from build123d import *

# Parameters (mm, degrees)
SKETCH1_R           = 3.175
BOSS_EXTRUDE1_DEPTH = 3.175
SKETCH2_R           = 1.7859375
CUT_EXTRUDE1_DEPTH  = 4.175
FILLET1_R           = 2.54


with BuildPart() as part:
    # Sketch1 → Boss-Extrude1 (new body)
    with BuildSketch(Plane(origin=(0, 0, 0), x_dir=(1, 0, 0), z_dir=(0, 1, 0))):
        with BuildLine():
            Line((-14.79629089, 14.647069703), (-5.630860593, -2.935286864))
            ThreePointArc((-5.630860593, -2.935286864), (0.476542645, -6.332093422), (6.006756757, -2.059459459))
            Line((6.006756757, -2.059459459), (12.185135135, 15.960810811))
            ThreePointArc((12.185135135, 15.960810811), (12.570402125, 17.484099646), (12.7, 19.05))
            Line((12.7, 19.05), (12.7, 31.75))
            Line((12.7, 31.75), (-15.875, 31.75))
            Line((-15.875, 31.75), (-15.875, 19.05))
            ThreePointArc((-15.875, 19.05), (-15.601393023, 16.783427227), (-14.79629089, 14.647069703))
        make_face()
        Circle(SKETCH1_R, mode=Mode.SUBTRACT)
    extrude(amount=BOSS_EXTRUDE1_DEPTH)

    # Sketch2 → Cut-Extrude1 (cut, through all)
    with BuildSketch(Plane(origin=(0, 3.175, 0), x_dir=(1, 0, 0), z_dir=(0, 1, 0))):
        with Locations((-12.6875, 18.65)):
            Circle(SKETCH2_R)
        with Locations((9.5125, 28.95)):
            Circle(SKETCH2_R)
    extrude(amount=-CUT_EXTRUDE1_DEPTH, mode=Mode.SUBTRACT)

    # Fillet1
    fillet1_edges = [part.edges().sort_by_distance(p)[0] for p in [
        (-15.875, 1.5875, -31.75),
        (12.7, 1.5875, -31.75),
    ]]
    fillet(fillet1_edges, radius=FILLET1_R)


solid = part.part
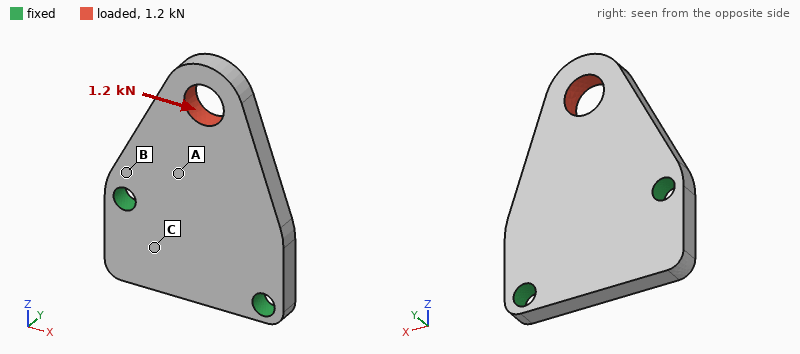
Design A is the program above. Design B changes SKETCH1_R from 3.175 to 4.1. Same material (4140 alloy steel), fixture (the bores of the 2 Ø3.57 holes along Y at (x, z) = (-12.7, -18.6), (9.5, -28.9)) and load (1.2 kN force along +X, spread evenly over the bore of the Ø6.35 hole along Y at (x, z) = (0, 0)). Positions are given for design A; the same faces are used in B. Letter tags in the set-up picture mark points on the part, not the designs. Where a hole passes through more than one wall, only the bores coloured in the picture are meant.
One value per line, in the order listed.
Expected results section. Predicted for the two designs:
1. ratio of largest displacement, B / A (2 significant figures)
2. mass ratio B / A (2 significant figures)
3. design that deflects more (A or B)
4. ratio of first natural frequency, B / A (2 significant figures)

1.4
0.97
B
1.1
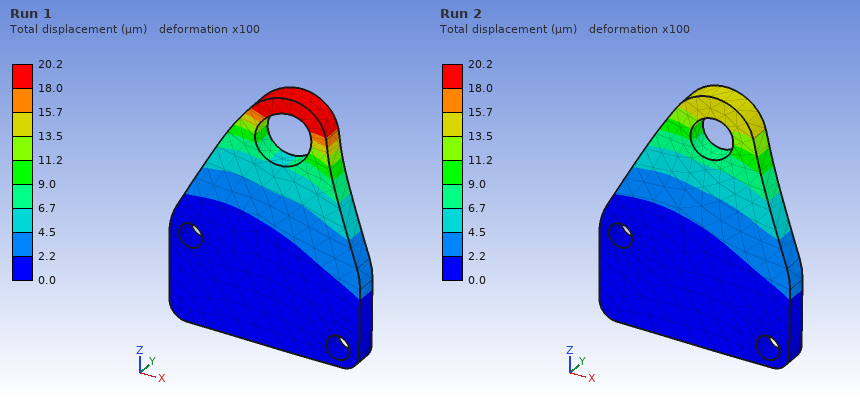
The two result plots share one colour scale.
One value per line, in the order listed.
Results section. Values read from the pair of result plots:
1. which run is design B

Run 1
